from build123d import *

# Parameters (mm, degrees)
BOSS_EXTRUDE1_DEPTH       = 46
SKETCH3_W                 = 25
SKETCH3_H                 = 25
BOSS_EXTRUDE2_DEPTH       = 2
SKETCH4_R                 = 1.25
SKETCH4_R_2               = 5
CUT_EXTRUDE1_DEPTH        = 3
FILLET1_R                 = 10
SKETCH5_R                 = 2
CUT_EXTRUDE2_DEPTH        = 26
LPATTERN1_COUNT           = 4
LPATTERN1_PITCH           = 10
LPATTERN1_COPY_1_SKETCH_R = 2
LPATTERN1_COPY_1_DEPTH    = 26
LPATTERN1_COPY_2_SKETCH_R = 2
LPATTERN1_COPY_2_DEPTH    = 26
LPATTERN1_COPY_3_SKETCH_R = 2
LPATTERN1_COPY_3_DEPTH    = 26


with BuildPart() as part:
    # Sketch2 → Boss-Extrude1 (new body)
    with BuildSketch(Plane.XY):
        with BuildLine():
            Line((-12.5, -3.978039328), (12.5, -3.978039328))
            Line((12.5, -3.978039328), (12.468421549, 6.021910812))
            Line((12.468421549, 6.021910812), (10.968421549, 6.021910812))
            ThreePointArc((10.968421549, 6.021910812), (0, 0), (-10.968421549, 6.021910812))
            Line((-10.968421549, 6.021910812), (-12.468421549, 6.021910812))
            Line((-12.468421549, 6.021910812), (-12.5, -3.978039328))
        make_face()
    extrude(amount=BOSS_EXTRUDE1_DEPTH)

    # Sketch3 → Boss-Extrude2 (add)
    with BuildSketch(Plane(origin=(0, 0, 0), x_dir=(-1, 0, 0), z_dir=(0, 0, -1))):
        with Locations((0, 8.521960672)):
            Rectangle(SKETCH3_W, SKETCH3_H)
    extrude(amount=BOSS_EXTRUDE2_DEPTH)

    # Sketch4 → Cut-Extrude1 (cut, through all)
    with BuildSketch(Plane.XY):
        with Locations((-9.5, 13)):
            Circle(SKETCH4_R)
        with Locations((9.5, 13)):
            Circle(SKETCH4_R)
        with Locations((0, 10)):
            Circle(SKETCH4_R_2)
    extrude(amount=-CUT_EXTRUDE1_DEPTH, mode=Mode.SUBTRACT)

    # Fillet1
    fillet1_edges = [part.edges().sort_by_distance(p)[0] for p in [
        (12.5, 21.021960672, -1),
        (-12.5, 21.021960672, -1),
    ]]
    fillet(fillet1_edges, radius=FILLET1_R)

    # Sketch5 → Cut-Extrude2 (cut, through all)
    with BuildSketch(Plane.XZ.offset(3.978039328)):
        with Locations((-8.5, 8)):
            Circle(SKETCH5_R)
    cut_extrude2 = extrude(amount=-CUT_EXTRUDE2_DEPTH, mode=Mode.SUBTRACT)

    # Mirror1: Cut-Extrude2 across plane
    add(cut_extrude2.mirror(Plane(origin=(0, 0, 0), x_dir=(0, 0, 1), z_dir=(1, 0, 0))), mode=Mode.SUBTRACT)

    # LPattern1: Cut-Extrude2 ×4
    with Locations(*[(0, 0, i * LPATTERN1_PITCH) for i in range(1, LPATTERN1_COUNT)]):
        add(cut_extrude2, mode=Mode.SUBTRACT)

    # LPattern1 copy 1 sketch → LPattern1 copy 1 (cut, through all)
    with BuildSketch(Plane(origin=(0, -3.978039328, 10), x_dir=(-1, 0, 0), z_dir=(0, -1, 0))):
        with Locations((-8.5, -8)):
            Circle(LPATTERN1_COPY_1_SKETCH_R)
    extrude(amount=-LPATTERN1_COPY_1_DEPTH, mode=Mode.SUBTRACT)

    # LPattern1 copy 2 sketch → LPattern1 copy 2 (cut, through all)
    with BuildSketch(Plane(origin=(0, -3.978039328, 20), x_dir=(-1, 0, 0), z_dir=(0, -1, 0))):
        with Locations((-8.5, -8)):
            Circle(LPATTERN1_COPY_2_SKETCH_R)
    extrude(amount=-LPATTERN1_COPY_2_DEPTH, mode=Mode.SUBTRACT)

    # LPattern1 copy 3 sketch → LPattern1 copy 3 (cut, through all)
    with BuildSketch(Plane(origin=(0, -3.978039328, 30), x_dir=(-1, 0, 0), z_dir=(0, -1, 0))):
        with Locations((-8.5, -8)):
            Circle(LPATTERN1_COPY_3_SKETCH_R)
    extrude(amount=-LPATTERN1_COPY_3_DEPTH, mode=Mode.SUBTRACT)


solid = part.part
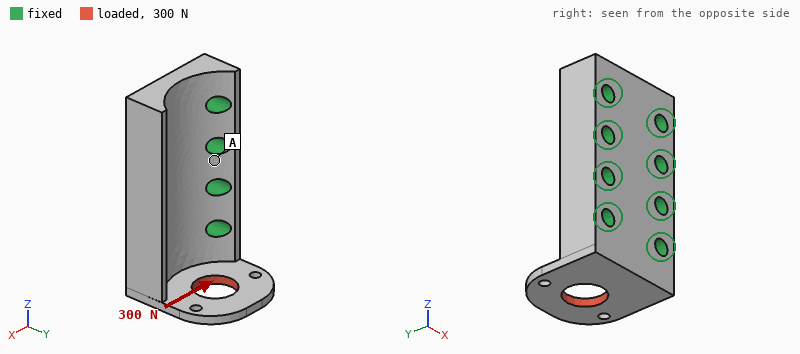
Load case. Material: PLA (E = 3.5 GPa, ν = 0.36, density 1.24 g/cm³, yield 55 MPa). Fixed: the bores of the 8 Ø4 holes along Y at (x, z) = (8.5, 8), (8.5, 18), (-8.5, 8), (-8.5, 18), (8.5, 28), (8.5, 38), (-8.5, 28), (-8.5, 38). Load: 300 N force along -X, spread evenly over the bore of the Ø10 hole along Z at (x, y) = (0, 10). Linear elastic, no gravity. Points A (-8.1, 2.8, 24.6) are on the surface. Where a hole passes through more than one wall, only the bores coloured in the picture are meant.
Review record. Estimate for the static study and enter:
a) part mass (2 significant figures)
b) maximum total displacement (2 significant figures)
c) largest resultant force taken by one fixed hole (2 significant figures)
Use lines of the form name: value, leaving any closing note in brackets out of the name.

part mass: 9.3 g
maximum total displacement: 0.25 mm
largest resultant force taken by one fixed hole: 230 N
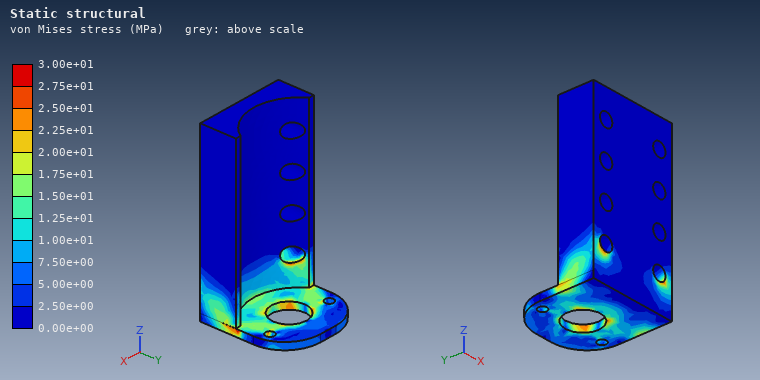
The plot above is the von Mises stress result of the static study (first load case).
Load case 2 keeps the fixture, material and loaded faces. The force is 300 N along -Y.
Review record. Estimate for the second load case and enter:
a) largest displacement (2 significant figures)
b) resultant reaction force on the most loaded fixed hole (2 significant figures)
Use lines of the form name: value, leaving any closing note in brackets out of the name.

largest displacement: 0.16 mm
resultant reaction force on the most loaded fixed hole: 160 N
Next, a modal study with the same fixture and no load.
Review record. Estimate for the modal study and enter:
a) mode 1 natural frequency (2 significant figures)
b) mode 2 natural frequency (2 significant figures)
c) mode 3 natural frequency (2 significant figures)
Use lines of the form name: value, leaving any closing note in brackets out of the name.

mode 1 natural frequency: 1700 Hz
mode 2 natural frequency: 4200 Hz
mode 3 natural frequency: 6600 Hz
